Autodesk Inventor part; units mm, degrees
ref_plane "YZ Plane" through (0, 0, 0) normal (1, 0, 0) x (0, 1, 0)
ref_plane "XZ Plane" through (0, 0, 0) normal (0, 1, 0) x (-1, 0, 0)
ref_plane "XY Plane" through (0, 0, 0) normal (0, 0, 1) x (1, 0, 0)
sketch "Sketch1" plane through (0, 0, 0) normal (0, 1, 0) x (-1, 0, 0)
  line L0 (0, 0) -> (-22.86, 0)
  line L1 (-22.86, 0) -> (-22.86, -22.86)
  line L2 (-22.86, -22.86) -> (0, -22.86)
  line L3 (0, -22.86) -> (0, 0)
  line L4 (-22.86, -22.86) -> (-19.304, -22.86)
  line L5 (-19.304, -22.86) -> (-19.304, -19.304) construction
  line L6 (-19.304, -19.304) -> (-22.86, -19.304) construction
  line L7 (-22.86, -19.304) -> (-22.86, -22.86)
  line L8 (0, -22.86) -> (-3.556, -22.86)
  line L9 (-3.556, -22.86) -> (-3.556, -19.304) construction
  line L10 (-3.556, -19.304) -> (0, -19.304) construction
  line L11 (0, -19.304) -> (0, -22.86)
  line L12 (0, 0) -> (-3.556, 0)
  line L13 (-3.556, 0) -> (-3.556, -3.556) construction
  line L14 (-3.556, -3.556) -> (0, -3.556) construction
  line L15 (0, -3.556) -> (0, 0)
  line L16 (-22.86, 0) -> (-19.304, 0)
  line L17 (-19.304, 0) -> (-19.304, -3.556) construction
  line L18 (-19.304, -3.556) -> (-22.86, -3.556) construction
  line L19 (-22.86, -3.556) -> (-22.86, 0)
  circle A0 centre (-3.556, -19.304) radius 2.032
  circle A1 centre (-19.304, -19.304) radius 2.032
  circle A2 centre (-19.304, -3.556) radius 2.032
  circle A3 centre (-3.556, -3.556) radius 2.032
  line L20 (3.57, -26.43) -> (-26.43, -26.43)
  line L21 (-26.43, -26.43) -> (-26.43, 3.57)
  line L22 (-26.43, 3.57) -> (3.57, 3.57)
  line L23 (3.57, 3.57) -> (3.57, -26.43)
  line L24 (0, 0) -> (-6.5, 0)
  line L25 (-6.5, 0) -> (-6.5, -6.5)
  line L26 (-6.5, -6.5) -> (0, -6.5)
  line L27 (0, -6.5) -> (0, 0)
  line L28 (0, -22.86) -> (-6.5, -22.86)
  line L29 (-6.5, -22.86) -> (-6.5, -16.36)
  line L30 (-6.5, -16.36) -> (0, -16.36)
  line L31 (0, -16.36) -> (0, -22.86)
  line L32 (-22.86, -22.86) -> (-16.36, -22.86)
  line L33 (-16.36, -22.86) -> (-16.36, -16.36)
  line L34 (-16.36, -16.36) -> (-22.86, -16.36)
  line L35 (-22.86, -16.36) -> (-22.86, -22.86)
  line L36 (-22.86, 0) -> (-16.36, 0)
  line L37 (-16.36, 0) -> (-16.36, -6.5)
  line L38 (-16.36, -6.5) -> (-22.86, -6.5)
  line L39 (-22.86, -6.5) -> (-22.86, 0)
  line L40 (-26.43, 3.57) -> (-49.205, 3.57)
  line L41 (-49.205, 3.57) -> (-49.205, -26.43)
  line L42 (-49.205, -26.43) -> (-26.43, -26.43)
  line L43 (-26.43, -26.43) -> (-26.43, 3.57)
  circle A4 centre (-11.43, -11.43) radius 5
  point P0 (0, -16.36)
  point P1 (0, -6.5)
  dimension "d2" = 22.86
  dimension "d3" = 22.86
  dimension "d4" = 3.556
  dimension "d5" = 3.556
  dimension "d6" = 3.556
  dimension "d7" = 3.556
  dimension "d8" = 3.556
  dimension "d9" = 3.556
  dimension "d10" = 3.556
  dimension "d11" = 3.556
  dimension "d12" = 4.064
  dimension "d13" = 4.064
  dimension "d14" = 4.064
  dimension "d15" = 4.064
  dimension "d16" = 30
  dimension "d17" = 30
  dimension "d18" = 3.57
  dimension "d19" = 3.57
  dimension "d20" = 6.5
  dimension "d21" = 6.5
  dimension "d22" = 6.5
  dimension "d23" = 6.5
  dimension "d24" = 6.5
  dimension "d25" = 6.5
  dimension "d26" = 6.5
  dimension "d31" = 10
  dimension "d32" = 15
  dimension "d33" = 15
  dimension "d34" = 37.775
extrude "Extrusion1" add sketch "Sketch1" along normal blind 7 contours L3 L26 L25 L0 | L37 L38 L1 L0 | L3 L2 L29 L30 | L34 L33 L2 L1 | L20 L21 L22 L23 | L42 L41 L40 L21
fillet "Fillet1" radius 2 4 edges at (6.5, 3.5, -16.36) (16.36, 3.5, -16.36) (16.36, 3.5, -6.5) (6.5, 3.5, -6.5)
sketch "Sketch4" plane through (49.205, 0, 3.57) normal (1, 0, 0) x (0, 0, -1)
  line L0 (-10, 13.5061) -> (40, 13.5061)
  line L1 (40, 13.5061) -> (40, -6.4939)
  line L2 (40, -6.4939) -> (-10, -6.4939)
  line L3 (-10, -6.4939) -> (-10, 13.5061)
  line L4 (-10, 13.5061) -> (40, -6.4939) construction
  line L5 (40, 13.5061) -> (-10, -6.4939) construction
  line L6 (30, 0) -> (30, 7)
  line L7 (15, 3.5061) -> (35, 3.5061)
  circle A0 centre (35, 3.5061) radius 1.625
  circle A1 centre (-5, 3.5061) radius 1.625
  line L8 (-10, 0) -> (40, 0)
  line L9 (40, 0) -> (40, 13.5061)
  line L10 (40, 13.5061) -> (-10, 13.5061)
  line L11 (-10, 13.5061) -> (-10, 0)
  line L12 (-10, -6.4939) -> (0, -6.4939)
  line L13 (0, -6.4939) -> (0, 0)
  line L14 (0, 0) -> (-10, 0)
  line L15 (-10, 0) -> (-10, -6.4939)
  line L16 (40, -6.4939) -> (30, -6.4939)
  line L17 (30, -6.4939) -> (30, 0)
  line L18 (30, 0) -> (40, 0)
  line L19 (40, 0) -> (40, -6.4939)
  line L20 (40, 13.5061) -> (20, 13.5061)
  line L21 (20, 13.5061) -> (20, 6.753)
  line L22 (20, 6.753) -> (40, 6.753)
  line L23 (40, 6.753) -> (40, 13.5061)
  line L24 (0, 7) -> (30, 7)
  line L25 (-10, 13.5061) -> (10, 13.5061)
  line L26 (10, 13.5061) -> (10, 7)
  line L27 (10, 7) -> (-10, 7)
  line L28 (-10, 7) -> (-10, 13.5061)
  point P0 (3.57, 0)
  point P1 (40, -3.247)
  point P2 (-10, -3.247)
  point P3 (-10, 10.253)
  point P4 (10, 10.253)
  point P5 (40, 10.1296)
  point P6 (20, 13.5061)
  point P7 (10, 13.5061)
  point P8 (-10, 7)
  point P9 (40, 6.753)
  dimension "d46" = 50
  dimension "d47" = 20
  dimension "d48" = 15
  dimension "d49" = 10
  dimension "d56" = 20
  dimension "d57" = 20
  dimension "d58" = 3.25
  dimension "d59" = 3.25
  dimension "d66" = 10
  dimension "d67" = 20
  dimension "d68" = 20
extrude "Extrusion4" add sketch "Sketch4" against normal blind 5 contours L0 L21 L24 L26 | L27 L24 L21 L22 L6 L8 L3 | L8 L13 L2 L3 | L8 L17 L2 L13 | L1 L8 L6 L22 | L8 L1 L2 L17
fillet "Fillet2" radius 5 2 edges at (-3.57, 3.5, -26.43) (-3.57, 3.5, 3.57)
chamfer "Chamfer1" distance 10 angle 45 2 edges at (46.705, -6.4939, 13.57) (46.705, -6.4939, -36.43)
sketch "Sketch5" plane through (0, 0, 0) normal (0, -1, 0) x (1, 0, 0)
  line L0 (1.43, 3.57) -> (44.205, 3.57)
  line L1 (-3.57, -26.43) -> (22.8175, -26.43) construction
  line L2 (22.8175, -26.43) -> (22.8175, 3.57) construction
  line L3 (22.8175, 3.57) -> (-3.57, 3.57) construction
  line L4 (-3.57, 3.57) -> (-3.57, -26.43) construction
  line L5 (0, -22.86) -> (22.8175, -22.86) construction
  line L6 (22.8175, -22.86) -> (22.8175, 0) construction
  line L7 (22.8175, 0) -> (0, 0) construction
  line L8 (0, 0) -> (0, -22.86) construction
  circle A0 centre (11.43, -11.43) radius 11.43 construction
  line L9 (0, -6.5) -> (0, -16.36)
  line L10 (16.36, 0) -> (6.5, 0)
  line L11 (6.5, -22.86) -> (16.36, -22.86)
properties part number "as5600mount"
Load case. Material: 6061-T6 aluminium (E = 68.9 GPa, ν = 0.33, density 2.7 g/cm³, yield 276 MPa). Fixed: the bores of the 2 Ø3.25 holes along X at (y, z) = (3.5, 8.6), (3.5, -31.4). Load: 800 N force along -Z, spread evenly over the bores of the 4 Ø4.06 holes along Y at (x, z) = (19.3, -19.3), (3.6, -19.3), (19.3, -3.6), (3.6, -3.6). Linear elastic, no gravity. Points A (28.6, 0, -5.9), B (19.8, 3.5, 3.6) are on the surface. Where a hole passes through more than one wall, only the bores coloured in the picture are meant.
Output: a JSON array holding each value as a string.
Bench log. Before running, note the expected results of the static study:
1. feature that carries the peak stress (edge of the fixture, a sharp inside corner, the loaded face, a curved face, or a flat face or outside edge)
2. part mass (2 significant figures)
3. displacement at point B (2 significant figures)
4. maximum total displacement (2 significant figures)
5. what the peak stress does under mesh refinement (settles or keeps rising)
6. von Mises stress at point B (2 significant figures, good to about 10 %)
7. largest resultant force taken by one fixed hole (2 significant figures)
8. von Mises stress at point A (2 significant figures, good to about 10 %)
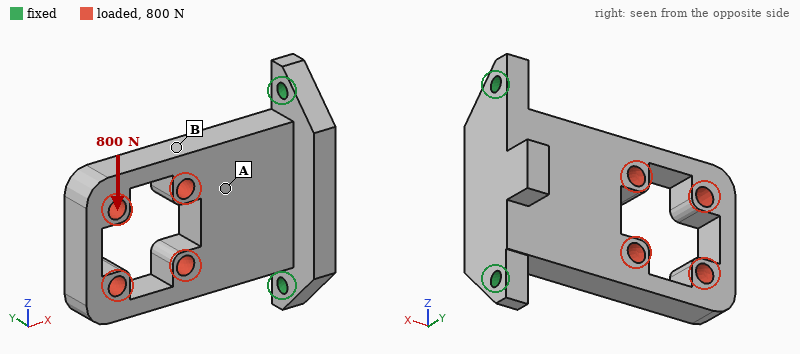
["edge of the fixture", "28 g", "0.034 mm", "0.11 mm", "keeps rising", "51 MPa", "930 N", "13 MPa"]
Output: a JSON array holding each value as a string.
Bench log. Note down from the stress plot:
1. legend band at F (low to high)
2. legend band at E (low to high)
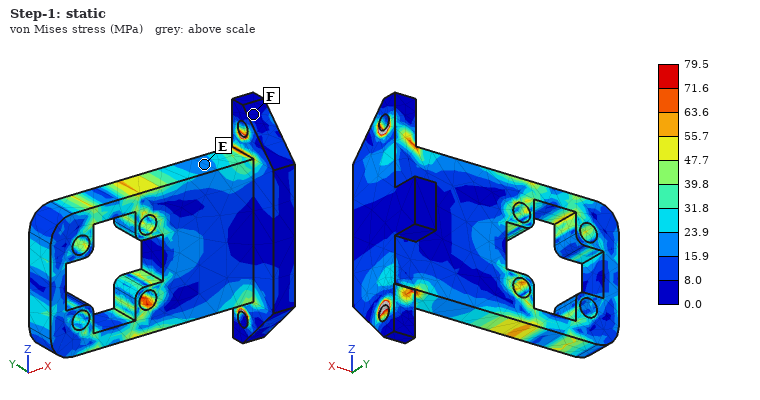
["0.0 to 8.0 MPa", "15.9 to 23.9 MPa"]
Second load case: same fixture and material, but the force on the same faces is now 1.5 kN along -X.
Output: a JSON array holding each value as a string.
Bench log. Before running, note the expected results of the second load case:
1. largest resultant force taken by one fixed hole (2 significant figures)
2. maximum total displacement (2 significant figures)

["800 N", "40 µm"]
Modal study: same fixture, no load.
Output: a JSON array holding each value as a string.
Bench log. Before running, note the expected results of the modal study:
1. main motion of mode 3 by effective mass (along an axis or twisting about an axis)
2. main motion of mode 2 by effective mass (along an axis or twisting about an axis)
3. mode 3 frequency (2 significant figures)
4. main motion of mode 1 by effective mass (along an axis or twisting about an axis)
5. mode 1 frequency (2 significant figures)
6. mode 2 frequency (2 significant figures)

["twisting about X", "along Z", "5900 Hz", "along Y", "1700 Hz", "5100 Hz"]
